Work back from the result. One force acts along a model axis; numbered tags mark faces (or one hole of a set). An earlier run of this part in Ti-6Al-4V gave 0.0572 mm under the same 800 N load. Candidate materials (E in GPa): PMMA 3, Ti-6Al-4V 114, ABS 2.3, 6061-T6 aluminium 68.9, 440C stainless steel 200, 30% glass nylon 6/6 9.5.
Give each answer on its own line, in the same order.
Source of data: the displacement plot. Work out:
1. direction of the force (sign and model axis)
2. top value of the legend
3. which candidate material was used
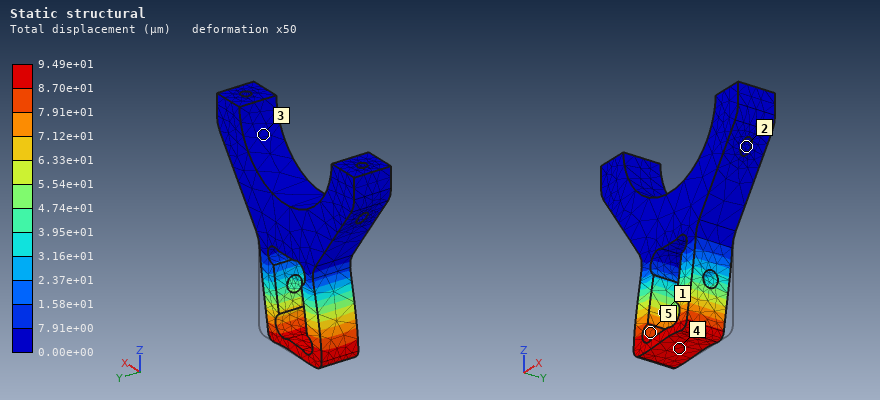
-X
9.49e+01 µm
6061-T6 aluminium
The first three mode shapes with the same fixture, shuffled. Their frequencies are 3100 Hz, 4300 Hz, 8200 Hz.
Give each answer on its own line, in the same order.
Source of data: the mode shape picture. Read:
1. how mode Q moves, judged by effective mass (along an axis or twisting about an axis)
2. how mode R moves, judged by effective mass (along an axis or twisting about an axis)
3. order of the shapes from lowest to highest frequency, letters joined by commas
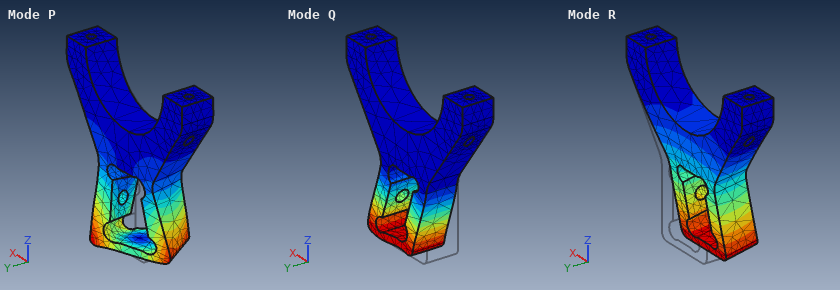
along X
along Y
R, Q, P
